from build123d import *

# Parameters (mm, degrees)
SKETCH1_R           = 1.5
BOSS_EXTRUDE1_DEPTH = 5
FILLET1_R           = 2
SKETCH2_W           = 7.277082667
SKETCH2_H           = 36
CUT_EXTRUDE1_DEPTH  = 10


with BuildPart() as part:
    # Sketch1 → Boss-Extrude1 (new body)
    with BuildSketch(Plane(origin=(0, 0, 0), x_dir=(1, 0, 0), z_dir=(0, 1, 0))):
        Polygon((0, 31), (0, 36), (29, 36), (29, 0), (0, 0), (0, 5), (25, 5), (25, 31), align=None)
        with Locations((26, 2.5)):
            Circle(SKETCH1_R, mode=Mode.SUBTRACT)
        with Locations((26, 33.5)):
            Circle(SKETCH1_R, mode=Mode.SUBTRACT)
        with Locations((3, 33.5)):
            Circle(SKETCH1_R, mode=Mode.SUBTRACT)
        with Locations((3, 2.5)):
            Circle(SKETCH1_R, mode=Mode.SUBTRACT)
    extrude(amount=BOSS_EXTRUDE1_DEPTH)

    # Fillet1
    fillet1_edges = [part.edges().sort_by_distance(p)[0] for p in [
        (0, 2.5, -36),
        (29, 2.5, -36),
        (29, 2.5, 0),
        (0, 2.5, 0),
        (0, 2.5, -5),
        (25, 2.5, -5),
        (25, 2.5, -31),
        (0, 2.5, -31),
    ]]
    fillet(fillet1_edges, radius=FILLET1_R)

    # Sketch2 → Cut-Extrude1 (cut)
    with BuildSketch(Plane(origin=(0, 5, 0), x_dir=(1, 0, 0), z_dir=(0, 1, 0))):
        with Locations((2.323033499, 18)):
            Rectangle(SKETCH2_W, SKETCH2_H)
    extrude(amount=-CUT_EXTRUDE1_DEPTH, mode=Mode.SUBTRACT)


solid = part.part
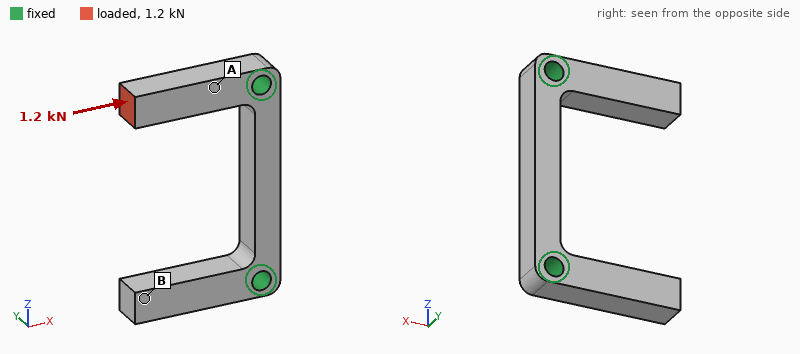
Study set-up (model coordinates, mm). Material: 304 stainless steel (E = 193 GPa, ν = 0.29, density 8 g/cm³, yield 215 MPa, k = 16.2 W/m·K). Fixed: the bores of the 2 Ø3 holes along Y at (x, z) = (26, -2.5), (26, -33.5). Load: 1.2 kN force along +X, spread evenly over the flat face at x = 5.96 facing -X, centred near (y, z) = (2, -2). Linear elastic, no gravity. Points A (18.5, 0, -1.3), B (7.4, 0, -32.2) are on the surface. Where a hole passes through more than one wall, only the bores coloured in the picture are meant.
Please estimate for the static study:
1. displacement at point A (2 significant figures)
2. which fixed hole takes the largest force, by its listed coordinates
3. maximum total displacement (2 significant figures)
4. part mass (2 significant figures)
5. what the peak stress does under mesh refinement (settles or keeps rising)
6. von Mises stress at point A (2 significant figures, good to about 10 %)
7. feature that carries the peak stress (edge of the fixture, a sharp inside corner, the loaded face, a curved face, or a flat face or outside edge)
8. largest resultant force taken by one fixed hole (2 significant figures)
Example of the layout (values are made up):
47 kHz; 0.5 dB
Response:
1.7 µm; (26, -2.5); 4.8 µm; 13 g; keeps rising; 48 MPa; edge of the fixture; 1.2 kN
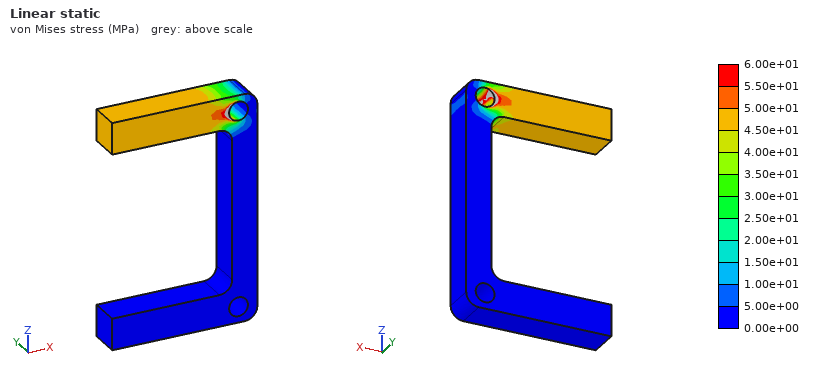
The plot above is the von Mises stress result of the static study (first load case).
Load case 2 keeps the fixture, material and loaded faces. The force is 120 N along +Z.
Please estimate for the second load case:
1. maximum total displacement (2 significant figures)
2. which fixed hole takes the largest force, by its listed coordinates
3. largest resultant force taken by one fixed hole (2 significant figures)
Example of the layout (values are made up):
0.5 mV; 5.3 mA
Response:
31 µm; (26, -2.5); 120 N
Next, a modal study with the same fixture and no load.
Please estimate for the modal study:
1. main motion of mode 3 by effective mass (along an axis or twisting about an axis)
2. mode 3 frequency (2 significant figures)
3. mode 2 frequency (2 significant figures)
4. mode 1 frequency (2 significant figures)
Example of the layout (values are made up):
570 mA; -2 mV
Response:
along Y; 10 kHz; 10000 Hz; 9900 Hz
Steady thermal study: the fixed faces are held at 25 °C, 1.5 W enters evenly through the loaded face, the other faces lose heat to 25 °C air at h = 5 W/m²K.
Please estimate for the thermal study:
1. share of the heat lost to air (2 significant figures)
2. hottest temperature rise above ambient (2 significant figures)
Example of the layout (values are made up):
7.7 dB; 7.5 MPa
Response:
4.3 %; 68 K
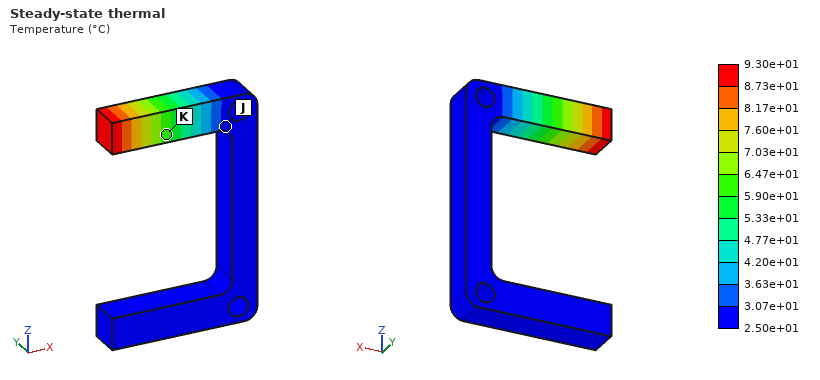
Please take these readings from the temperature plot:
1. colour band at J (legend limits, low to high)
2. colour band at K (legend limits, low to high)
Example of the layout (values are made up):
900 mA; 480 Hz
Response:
2.50e+01 to 3.07e+01 °C; 5.90e+01 to 6.47e+01 °C
